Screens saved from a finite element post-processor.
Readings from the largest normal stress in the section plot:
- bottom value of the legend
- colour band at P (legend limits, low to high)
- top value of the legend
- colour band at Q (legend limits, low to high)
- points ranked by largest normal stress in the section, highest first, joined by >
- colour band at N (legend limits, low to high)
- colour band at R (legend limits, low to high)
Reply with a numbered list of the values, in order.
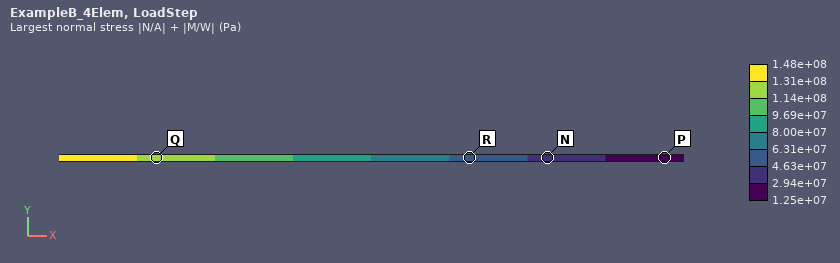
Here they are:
1. 1.25e+07 Pa
2. 1.25e+07 to 2.94e+07 Pa
3. 1.48e+08 Pa
4. 1.14e+08 to 1.31e+08 Pa
5. Q > R > N > P
6. 2.94e+07 to 4.63e+07 Pa
7. 4.63e+07 to 6.31e+07 Pa
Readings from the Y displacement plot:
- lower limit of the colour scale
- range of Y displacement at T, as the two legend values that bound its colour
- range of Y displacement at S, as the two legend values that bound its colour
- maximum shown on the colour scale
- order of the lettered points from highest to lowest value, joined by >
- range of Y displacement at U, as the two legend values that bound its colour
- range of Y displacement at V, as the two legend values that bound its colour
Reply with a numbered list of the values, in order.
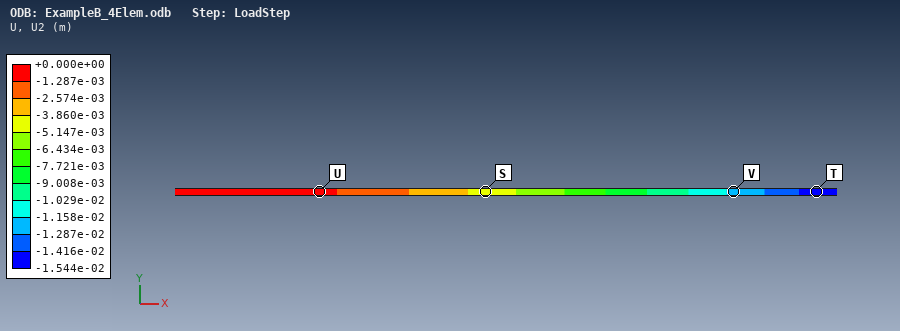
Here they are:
1. -1.544e-02 m
2. -1.544e-02 to -1.416e-02 m
3. -5.147e-03 to -3.860e-03 m
4. +0.000e+00 m
5. U > S > V > T
6. -1.287e-03 to +0.000e+00 m
7. -1.287e-02 to -1.158e-02 m
